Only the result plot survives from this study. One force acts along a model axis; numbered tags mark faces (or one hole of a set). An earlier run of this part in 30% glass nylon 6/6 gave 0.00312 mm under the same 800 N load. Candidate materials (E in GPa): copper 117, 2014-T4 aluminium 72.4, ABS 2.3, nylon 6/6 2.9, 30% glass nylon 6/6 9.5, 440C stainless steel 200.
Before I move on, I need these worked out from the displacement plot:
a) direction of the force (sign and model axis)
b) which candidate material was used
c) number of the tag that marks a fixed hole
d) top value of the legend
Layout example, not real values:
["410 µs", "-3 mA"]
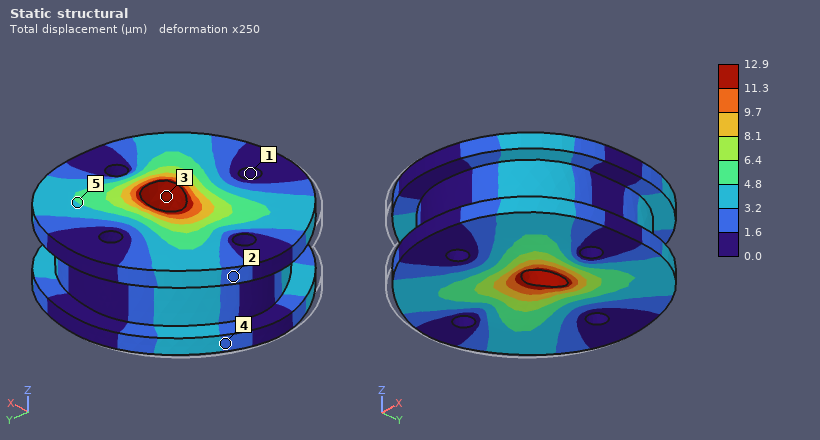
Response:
["+X", "ABS", "1", "12.9 µm"]
